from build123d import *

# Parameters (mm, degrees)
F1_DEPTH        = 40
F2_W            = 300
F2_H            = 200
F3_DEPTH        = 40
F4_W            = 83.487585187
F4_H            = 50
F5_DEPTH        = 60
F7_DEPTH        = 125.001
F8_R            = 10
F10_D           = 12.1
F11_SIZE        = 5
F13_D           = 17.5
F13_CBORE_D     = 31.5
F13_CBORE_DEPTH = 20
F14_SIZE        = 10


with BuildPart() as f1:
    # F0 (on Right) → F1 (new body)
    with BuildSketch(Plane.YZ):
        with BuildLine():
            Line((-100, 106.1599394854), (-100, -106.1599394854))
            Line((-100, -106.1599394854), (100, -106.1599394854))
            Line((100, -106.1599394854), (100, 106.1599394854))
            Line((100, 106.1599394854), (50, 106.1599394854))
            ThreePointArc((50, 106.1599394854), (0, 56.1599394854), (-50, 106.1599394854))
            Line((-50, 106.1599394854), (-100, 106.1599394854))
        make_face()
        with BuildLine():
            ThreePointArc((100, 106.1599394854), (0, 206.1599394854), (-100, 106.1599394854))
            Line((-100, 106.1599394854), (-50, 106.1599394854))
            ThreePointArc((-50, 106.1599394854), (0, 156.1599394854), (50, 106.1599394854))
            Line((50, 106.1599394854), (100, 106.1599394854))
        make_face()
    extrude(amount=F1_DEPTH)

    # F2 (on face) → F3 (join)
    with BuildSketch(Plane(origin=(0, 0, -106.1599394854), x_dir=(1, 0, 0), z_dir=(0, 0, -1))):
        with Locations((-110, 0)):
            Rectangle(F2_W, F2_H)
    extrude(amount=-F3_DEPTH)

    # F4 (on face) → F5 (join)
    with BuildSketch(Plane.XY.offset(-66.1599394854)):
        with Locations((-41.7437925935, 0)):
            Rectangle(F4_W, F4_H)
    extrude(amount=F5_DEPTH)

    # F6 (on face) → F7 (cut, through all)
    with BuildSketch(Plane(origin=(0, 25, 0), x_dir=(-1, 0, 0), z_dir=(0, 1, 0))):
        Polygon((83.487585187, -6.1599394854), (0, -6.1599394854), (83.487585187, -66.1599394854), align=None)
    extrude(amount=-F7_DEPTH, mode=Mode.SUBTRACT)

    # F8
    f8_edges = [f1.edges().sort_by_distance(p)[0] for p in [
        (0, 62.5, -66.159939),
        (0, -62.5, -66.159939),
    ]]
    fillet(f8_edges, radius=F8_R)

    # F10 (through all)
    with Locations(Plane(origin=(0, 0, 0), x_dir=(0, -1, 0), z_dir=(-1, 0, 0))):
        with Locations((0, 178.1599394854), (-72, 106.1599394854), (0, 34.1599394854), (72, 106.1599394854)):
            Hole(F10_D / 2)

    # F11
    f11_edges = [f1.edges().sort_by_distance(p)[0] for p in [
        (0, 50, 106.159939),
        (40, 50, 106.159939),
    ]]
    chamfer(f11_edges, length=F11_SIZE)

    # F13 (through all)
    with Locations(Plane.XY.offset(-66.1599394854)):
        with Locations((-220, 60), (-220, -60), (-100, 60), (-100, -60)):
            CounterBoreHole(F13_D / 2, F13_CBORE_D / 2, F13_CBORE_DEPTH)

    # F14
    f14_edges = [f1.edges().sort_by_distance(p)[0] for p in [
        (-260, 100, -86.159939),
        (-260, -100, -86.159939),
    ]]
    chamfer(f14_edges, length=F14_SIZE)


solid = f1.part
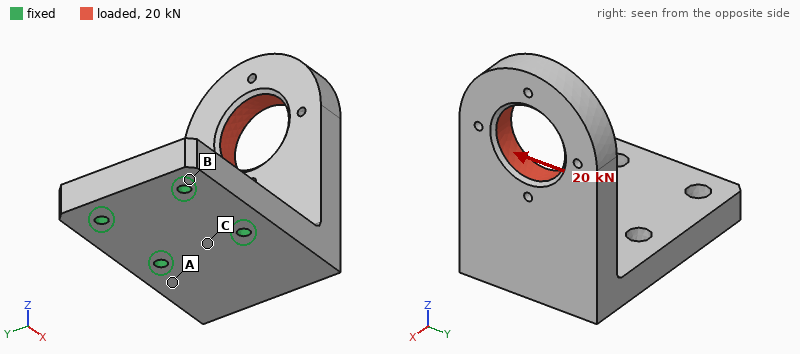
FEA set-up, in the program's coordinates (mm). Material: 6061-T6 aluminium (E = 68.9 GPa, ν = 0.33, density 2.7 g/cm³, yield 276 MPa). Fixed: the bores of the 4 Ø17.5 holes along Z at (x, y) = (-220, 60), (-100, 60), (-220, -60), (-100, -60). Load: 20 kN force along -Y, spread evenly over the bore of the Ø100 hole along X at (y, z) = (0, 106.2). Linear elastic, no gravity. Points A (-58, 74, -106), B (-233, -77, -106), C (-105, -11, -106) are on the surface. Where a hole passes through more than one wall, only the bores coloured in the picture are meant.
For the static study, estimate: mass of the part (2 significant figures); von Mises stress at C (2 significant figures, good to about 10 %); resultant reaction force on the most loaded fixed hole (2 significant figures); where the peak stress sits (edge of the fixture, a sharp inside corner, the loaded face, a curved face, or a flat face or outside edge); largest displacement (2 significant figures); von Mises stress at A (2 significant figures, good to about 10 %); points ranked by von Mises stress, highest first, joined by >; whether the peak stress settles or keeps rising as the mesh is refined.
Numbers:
11 kg
15 MPa
41 kN
edge of the fixture
0.71 mm
27 MPa
A > C > B
keeps rising
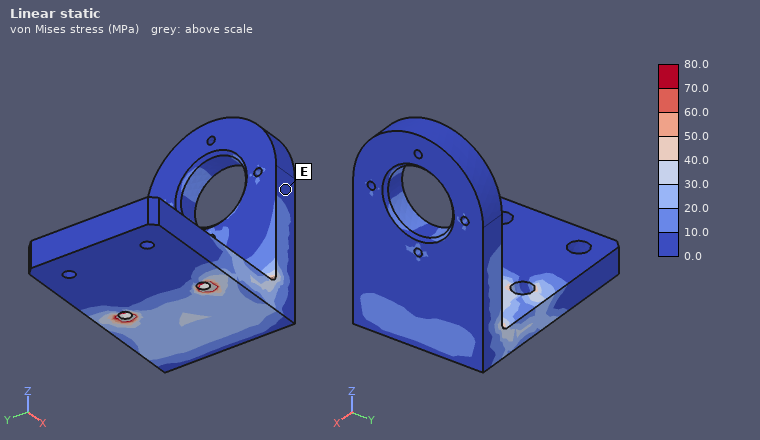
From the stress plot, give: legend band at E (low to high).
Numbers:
0.0 to 10.0 MPa
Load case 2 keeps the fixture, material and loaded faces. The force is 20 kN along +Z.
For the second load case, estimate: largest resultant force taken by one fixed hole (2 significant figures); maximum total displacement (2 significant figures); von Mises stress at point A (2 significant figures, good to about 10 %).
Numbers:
21 kN
0.75 mm
25 MPa
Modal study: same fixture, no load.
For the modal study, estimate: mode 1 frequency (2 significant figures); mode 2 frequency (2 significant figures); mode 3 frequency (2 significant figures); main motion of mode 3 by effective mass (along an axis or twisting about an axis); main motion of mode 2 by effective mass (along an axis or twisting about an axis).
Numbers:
320 Hz
560 Hz
950 Hz
along Z
along Y
